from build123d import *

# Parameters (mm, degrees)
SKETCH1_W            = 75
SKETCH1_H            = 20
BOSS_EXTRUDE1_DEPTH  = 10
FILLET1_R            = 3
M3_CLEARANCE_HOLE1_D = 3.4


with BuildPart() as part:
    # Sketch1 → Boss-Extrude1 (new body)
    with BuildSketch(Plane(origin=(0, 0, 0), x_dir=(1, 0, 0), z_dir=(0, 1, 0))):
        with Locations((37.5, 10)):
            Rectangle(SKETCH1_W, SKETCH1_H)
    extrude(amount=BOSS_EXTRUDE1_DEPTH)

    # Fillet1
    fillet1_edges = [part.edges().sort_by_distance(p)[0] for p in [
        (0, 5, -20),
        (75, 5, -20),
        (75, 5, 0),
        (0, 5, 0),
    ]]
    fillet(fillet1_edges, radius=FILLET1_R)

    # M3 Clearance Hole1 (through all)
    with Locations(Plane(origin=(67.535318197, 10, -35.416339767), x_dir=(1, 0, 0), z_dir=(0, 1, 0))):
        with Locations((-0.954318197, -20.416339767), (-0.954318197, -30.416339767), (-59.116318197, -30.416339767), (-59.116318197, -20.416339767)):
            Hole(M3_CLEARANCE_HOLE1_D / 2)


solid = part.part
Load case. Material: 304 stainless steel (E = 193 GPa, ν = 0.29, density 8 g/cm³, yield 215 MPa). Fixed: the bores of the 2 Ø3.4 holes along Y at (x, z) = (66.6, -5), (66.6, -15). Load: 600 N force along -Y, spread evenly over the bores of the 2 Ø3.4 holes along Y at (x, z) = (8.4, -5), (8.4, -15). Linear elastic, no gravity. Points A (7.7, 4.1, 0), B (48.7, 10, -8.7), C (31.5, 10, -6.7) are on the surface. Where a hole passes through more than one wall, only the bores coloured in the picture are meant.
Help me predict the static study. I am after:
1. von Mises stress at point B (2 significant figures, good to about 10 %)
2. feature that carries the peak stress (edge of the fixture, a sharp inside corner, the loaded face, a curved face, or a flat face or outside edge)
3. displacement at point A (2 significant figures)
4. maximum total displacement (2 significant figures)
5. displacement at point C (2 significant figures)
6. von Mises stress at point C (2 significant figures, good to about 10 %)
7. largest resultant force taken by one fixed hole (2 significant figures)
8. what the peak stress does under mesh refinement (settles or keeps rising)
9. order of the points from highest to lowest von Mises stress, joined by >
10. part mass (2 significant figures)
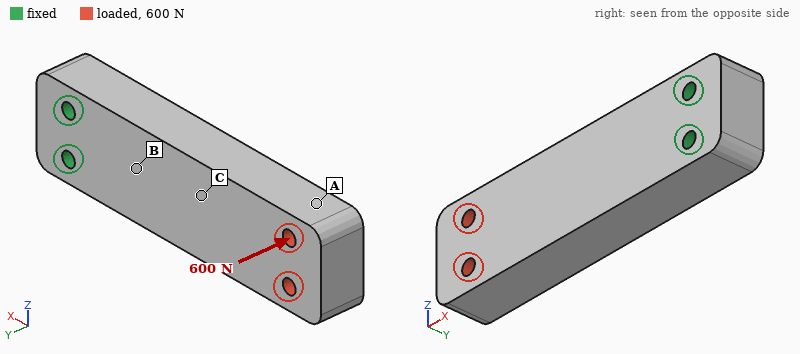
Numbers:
72 MPa
edge of the fixture
0.13 mm
0.15 mm
0.056 mm
42 MPa
300 N
keeps rising
B > C > A
120 g
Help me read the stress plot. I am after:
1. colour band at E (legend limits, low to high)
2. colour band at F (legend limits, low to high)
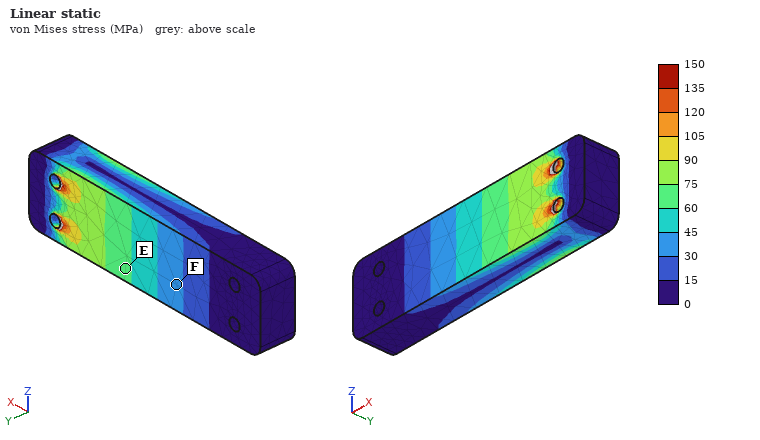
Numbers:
60 to 75 MPa
30 to 45 MPa
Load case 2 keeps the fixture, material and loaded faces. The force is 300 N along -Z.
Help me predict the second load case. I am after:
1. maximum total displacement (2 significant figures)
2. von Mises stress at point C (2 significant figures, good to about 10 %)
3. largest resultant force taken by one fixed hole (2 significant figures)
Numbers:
21 µm
5.0 MPa
1.5 kN
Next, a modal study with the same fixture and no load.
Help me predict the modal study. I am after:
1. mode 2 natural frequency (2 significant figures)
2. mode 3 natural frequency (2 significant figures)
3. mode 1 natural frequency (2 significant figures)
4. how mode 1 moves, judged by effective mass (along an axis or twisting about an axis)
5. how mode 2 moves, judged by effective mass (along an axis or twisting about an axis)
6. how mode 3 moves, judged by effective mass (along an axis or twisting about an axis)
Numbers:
3300 Hz
9000 Hz
1800 Hz
along Y
along Z
twisting about X
